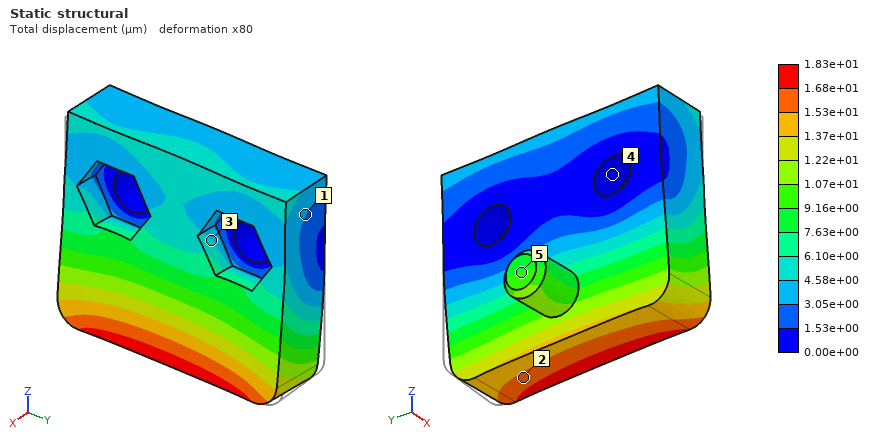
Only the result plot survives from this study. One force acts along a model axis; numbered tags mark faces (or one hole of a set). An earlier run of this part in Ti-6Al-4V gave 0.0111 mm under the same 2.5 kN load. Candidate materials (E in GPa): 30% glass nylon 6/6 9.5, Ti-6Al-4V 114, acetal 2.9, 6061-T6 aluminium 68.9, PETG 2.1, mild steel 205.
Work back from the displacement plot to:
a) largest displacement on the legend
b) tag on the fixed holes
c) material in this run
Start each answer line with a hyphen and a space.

- 1.83e+01 µm
- 4
- 6061-T6 aluminium
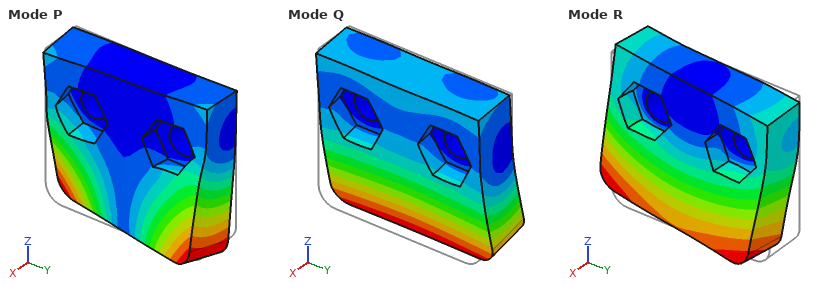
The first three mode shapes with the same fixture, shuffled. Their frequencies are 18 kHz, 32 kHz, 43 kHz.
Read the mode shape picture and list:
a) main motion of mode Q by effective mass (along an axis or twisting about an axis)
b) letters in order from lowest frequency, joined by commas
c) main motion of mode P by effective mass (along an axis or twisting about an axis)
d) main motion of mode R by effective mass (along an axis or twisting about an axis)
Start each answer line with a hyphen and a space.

- along X
- Q, P, R
- twisting about Z
- along Y
